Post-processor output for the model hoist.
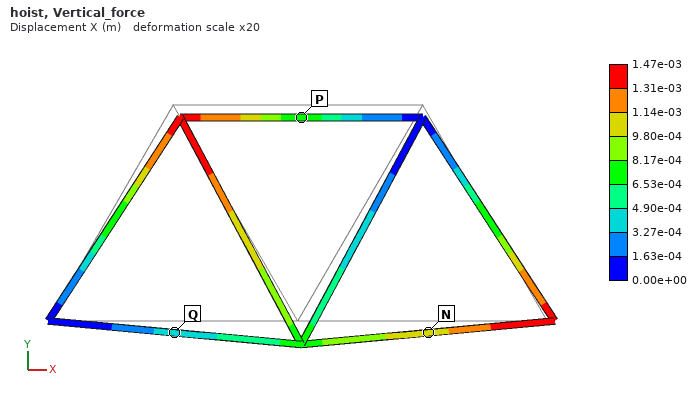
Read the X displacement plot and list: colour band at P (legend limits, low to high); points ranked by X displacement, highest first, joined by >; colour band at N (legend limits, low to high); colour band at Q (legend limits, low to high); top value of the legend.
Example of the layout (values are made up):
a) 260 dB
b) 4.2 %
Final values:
a) 6.53e-04 to 8.17e-04 m
b) N > P > Q
c) 9.80e-04 to 1.14e-03 m
d) 3.27e-04 to 4.90e-04 m
e) 1.47e-03 m
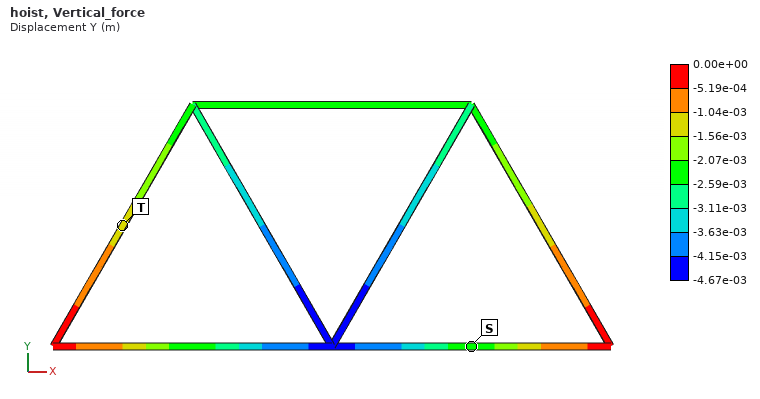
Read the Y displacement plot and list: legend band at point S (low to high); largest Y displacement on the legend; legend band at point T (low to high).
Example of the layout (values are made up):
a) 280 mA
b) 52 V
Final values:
a) -2.59e-03 to -2.07e-03 m
b) 0.00e+00 m
c) -1.56e-03 to -1.04e-03 m
